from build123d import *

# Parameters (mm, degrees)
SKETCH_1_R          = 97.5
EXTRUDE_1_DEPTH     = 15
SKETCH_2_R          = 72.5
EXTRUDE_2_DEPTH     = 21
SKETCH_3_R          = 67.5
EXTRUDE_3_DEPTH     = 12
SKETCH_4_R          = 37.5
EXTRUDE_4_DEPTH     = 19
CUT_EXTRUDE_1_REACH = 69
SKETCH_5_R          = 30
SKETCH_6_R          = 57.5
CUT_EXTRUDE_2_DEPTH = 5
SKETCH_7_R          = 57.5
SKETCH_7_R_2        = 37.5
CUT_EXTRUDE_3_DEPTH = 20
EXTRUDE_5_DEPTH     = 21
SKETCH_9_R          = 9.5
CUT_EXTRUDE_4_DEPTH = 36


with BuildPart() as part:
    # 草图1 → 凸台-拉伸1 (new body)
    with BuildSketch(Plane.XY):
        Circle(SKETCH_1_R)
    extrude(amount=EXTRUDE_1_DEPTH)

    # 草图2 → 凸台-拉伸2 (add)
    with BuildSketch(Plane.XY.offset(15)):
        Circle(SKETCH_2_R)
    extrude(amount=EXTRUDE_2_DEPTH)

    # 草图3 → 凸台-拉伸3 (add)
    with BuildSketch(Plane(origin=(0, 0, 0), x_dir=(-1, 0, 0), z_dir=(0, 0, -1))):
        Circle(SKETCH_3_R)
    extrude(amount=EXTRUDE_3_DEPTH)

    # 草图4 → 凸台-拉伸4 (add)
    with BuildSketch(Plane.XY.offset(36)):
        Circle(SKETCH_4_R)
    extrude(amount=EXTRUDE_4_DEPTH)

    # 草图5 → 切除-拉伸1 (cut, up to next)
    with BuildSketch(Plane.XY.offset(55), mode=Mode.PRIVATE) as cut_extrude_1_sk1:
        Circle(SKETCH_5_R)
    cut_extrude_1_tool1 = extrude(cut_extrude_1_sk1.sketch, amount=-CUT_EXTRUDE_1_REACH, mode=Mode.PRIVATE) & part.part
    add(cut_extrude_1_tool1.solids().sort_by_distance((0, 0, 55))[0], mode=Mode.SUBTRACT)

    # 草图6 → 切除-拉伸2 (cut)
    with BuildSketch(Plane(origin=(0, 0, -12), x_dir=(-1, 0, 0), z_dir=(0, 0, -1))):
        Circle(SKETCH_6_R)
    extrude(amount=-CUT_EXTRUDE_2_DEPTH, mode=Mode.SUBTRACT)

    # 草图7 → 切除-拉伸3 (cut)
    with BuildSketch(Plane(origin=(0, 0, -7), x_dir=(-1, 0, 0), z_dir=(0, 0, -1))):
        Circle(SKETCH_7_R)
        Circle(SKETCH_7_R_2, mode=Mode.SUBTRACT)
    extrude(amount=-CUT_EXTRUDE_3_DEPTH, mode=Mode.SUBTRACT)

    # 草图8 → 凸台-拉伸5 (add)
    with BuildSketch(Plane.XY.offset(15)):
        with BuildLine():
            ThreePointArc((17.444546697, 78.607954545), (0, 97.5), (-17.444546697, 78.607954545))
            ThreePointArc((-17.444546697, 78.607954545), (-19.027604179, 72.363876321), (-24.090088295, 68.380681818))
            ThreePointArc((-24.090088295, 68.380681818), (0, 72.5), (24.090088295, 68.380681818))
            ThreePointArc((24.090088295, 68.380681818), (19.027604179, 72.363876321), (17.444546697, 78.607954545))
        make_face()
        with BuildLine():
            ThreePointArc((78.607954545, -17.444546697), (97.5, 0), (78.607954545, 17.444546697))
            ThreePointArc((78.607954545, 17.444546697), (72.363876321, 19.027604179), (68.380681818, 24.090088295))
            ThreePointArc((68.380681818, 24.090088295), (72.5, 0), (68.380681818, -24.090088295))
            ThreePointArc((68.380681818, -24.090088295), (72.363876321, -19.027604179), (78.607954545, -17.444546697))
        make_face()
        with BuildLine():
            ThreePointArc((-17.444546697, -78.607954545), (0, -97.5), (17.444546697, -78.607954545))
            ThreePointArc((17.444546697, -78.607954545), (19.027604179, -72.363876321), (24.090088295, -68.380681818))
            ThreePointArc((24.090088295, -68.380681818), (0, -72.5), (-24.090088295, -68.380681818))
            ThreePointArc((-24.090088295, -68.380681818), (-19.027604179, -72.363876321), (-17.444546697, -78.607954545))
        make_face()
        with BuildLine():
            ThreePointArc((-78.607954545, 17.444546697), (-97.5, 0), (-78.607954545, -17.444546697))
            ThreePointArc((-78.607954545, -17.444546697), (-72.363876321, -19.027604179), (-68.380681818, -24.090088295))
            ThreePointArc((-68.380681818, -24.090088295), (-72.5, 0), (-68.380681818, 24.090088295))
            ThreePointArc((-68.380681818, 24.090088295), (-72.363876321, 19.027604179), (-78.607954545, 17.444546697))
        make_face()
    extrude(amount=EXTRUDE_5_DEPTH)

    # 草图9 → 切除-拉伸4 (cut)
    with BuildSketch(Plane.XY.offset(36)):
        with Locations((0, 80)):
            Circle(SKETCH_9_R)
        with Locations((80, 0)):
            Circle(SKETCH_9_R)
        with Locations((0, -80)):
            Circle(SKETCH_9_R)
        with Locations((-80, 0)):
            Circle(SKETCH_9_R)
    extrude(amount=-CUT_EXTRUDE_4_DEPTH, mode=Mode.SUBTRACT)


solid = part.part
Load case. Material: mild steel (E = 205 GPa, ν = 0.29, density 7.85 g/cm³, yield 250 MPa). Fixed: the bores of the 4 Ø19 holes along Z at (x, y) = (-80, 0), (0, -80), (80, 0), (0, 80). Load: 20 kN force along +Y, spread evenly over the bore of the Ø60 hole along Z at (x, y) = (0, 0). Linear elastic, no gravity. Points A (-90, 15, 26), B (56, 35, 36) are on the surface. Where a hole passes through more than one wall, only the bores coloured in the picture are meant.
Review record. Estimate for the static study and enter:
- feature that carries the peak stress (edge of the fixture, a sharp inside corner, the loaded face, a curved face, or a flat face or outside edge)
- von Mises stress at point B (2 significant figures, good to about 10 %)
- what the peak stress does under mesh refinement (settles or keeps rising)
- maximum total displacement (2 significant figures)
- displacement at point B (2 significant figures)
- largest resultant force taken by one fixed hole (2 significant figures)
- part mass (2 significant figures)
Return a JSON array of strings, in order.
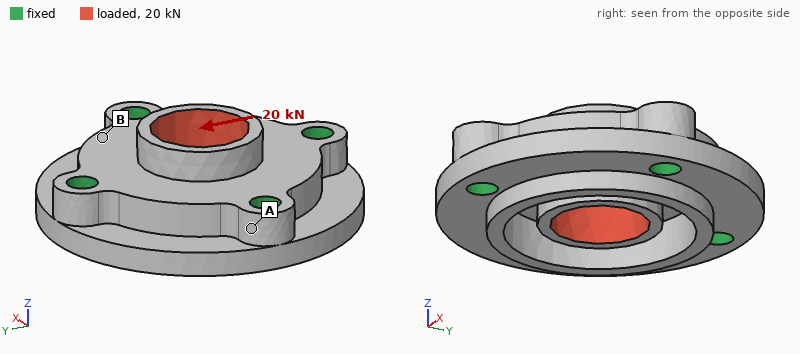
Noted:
["edge of the fixture", "2.0 MPa", "keeps rising", "3.8 µm", "1.00 µm", "6.4 kN", "5.7 kg"]
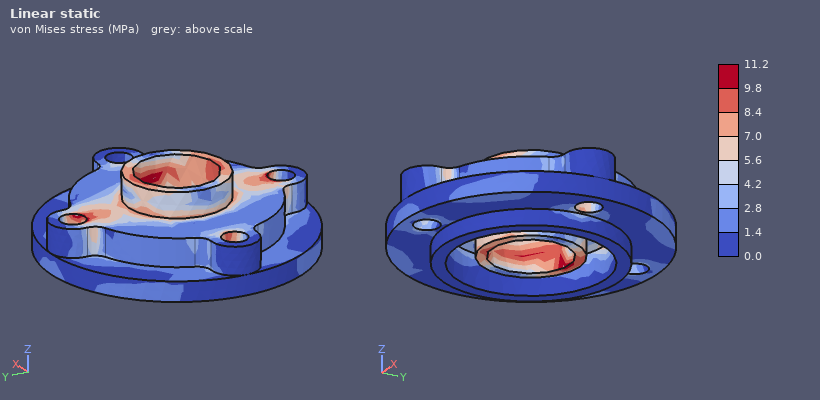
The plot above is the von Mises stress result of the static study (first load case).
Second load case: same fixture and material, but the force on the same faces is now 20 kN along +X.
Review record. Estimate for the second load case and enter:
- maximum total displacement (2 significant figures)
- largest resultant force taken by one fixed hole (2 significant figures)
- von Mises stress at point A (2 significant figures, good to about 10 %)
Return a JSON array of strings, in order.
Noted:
["3.7 µm", "6.4 kN", "1.5 MPa"]
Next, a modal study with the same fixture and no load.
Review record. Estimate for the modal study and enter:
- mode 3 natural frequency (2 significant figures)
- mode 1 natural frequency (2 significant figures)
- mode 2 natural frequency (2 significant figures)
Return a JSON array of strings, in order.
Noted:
["8000 Hz", "7400 Hz", "8000 Hz"]
